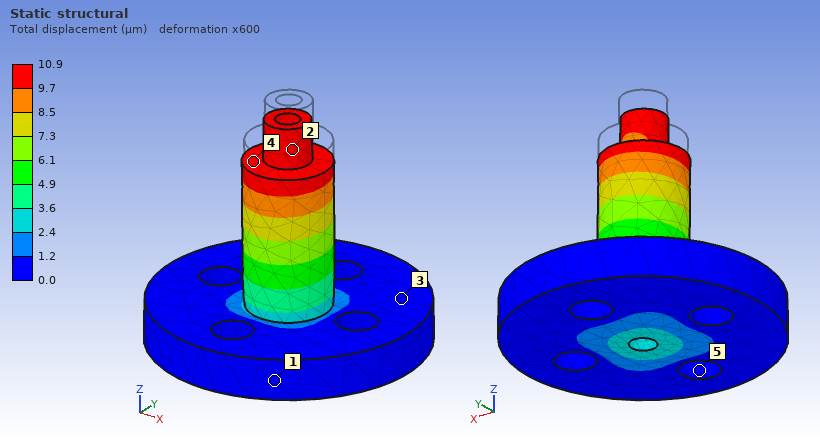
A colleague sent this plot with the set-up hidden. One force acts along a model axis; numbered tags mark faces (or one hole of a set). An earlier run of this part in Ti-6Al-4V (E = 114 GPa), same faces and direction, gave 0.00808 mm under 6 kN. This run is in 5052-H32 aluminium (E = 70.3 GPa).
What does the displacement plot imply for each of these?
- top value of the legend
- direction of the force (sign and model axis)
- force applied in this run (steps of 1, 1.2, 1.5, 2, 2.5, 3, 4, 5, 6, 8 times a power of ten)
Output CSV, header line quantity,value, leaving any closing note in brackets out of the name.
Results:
quantity,value
top value of the legend,10.9 µm
direction of the force,-Z
force applied in this run,5 kN
